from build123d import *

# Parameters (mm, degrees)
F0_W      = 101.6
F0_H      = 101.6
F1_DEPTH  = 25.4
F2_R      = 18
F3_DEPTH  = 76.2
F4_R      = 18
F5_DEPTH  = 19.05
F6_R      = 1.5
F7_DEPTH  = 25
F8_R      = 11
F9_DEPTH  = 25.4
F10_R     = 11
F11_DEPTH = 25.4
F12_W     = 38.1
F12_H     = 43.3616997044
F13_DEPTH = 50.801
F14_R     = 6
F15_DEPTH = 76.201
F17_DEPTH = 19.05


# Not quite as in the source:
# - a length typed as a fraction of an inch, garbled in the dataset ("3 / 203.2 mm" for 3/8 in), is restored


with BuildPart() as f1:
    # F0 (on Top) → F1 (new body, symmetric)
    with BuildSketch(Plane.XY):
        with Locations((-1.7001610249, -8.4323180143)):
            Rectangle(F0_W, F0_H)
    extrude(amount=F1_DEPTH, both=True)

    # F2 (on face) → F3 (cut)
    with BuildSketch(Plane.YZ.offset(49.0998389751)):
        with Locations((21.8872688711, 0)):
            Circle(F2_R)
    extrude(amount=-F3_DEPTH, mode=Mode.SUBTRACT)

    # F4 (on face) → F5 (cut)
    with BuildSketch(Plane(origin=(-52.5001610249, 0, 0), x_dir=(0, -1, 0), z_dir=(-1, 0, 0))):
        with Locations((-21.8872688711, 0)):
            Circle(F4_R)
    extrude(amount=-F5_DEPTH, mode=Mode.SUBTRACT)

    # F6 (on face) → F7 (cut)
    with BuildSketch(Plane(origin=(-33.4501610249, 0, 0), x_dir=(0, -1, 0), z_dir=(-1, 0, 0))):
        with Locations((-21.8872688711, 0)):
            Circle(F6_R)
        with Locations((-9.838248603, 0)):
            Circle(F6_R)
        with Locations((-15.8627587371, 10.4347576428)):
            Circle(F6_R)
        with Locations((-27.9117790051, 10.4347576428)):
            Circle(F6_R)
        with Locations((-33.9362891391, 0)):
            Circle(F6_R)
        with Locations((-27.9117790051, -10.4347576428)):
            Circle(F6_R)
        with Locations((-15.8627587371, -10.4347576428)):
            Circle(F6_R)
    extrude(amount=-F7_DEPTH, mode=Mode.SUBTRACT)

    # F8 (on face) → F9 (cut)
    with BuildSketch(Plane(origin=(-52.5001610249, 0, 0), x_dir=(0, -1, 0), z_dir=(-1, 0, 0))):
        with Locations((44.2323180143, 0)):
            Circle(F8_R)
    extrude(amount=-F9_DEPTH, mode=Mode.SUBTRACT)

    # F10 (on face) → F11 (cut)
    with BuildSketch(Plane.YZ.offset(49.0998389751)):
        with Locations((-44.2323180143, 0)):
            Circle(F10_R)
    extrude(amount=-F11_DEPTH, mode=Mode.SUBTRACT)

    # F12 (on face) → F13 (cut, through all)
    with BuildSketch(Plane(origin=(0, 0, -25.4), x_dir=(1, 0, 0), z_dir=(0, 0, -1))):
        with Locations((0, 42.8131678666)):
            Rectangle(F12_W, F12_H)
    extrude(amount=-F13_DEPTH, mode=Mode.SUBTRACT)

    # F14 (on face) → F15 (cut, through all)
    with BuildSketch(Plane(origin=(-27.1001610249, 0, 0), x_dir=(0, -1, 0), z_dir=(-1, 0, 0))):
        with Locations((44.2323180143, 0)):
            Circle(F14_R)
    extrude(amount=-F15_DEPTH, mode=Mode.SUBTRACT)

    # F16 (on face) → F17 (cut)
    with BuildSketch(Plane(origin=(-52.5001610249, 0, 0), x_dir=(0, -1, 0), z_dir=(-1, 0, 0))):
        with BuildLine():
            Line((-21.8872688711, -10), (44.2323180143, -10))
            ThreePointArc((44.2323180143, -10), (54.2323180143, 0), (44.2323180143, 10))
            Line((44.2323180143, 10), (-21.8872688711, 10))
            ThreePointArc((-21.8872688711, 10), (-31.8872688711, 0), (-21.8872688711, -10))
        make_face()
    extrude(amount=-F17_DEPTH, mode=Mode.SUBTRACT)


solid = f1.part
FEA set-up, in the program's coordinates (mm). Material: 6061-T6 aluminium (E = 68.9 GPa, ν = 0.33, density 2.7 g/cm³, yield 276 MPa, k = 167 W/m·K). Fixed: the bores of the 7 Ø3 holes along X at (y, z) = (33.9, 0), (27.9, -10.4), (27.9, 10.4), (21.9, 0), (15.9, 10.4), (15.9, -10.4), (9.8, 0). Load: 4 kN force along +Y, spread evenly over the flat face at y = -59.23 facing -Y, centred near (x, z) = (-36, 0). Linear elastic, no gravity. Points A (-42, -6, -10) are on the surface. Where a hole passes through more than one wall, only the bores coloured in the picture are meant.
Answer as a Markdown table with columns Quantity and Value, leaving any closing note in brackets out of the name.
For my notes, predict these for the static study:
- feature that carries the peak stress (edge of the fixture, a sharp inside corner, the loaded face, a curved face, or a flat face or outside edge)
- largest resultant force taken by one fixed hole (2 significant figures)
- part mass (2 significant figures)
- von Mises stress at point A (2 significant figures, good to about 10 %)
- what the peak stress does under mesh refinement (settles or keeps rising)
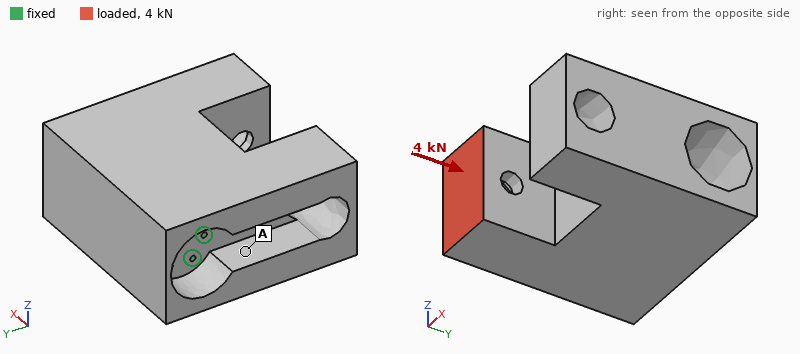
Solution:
| Quantity | Value |
|---|---|
| feature that carries the peak stress | edge of the fixture |
| largest resultant force taken by one fixed hole | 1.0 kN |
| part mass | 860 g |
| von Mises stress at point A | 2.5 MPa |
| what the peak stress does under mesh refinement | keeps rising |
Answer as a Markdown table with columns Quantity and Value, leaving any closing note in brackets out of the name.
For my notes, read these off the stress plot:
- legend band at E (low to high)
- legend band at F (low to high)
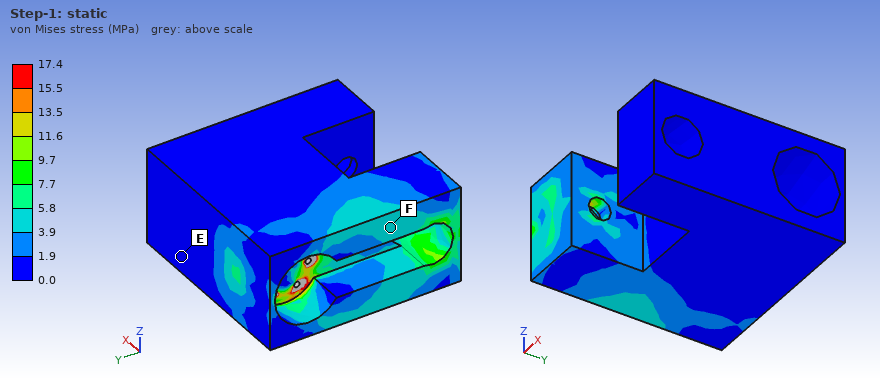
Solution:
| Quantity | Value |
|---|---|
| legend band at E | 0.0 to 1.9 MPa |
| legend band at F | 3.9 to 5.8 MPa |
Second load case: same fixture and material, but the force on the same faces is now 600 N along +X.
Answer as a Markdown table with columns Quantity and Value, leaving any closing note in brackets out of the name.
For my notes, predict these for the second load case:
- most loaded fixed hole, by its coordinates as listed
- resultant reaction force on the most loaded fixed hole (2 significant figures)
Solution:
| Quantity | Value |
|---|---|
| most loaded fixed hole, by its coordinates as listed | (9.8, 0) |
| resultant reaction force on the most loaded fixed hole | 1.1 kN |
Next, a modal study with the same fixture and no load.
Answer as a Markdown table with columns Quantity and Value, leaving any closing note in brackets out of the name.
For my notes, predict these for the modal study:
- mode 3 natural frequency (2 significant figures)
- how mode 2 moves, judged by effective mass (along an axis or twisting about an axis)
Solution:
| Quantity | Value |
|---|---|
| mode 3 natural frequency | 2600 Hz |
| how mode 2 moves, judged by effective mass | along Z |
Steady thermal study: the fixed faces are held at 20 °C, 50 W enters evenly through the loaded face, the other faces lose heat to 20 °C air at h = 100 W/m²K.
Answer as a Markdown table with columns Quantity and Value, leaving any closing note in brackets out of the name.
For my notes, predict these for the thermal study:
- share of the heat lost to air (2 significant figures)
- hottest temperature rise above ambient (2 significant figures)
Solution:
| Quantity | Value |
|---|---|
| share of the heat lost to air | 46 % |
| hottest temperature rise above ambient | 17 K |
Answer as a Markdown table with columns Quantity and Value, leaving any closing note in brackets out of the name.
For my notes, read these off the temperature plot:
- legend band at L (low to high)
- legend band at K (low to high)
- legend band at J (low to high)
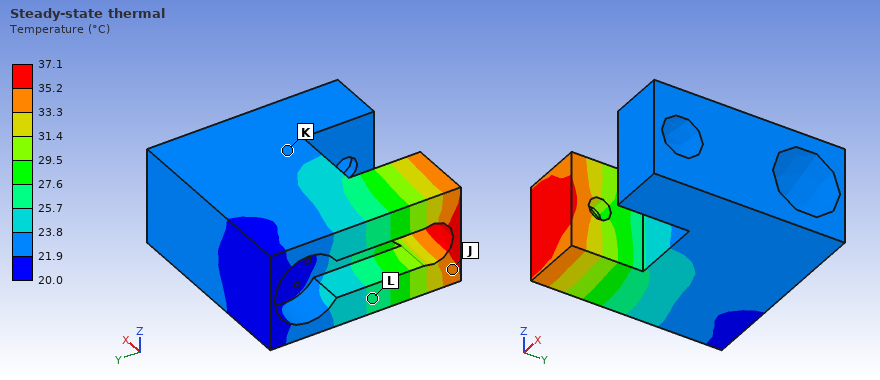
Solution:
| Quantity | Value |
|---|---|
| legend band at L | 25.7 to 27.6 °C |
| legend band at K | 21.9 to 23.8 °C |
| legend band at J | 33.3 to 35.2 °C |
